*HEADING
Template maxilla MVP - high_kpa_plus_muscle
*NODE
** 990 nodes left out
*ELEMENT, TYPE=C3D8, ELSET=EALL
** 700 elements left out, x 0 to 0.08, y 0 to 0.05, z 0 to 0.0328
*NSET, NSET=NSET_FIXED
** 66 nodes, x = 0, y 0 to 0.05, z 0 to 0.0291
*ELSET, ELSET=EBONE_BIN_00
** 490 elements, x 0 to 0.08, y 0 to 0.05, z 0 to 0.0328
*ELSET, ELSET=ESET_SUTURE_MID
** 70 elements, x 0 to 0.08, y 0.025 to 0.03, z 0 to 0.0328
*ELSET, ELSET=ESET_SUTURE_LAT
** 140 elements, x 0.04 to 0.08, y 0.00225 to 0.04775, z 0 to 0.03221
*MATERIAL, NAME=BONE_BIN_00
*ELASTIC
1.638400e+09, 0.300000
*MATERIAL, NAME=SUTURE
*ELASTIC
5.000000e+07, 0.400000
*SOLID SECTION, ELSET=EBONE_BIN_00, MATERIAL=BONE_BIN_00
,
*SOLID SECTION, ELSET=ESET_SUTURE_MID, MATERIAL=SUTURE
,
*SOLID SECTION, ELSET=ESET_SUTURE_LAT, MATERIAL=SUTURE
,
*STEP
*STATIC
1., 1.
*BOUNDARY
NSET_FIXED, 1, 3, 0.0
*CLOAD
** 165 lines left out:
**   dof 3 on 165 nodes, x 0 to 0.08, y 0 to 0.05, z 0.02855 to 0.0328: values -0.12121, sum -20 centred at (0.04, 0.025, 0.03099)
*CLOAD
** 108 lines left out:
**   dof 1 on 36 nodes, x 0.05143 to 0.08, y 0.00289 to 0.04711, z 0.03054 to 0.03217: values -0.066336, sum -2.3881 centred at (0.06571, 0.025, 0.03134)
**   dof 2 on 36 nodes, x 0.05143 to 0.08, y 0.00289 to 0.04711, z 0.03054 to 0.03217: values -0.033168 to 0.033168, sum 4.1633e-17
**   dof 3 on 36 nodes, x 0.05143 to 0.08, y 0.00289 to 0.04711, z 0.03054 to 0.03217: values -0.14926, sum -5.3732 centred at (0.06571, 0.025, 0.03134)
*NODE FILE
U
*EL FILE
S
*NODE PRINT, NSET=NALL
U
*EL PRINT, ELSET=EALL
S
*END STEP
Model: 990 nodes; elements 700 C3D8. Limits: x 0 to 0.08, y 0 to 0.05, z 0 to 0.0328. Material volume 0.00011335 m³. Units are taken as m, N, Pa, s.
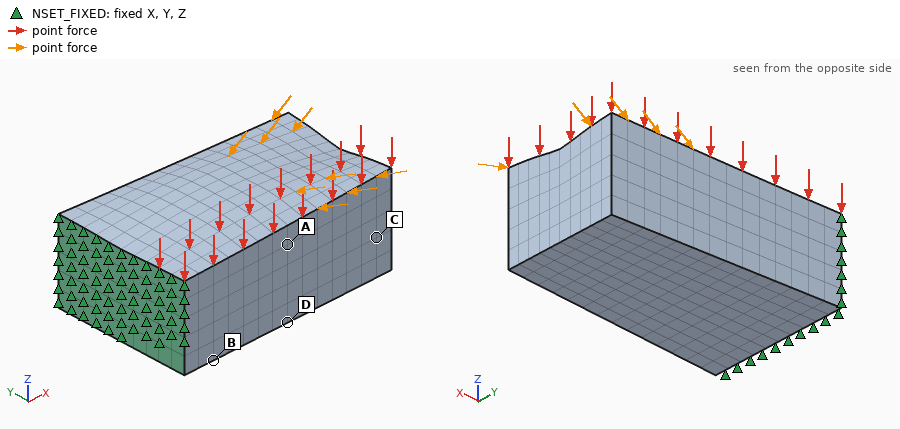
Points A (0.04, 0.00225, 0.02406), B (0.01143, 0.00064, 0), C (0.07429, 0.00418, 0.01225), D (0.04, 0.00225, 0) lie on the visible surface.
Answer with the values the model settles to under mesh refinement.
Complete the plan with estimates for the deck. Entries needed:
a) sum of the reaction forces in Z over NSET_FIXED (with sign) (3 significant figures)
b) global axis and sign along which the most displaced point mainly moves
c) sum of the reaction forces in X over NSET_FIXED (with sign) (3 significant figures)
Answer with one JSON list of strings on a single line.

["25.4 N", "-Z", "2.39 N"]
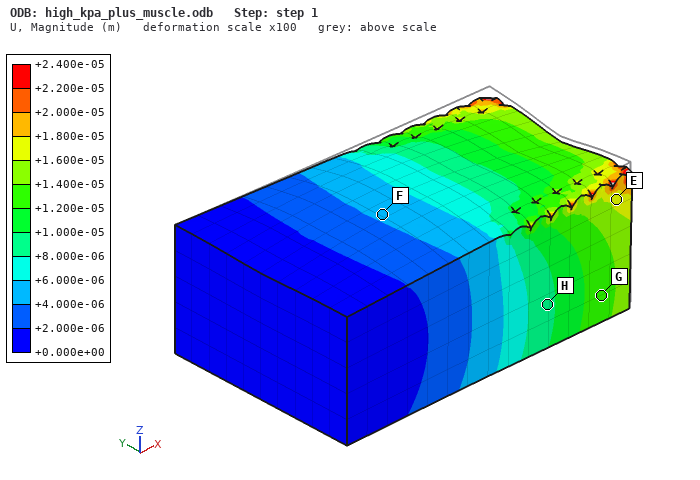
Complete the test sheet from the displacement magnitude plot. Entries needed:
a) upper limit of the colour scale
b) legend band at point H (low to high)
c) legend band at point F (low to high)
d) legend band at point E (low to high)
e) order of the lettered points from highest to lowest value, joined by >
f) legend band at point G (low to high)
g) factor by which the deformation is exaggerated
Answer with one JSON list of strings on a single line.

["+2.400e-05 m", "+8.000e-06 to +1.000e-05 m", "+4.000e-06 to +6.000e-06 m", "+1.600e-05 to +1.800e-05 m", "E > G > H > F", "+1.200e-05 to +1.400e-05 m", "100"]
